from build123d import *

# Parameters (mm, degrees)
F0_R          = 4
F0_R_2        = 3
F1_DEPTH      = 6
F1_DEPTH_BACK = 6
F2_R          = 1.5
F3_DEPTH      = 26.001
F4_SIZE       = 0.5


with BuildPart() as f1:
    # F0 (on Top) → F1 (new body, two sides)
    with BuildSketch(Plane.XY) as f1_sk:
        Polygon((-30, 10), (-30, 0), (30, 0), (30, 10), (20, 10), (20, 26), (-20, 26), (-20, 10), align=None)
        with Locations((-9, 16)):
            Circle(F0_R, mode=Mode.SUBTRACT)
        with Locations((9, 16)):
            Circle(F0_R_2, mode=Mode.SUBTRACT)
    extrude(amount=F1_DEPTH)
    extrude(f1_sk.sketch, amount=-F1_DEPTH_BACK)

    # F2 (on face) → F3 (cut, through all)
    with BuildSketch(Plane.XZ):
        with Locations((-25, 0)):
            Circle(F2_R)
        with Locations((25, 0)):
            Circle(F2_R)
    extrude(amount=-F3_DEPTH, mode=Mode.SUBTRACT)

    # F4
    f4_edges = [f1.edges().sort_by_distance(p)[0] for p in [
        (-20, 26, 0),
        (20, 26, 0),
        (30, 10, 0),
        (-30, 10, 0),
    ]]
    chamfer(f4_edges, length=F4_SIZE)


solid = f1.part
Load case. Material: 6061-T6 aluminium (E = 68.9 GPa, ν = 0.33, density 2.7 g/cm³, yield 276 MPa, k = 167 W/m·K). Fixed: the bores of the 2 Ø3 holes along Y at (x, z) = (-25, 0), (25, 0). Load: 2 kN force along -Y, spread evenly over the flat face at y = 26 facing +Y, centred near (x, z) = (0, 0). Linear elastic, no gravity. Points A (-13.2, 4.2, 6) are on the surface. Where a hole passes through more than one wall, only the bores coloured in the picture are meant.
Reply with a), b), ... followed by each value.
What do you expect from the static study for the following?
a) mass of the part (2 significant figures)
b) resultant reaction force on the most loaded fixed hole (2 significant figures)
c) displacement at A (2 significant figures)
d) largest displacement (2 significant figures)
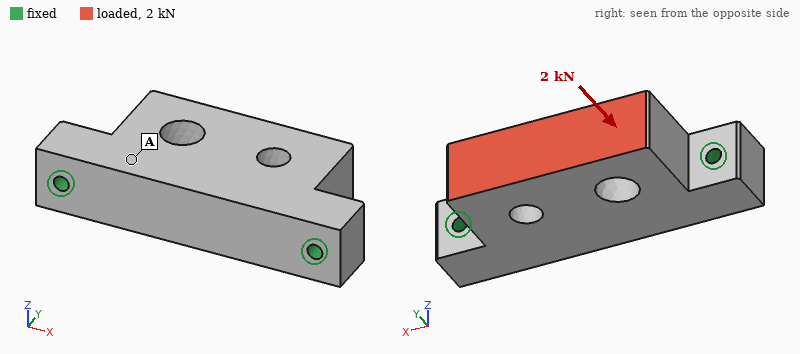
a) 37 g
b) 1.1 kN
c) 5.2 µm
d) 7.7 µm
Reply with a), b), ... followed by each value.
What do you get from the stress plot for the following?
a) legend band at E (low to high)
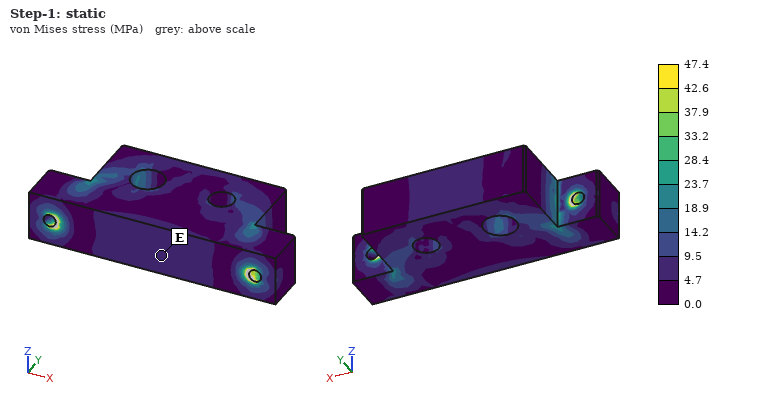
a) 4.7 to 9.5 MPa
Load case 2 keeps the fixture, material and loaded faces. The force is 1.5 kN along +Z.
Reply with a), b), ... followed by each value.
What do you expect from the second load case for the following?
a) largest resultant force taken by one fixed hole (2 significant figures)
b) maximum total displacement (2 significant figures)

a) 750 N
b) 84 µm
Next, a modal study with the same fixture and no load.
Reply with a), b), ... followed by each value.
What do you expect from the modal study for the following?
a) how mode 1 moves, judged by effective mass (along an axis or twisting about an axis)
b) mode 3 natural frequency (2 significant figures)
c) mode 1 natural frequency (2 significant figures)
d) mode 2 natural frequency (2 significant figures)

a) along Z
b) 16 kHz
c) 7200 Hz
d) 16 kHz
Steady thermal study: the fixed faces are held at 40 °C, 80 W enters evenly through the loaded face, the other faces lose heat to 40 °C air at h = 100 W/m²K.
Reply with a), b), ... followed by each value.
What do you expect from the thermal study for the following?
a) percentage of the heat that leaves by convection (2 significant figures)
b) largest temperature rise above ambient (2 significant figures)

a) 11 %
b) 41 K
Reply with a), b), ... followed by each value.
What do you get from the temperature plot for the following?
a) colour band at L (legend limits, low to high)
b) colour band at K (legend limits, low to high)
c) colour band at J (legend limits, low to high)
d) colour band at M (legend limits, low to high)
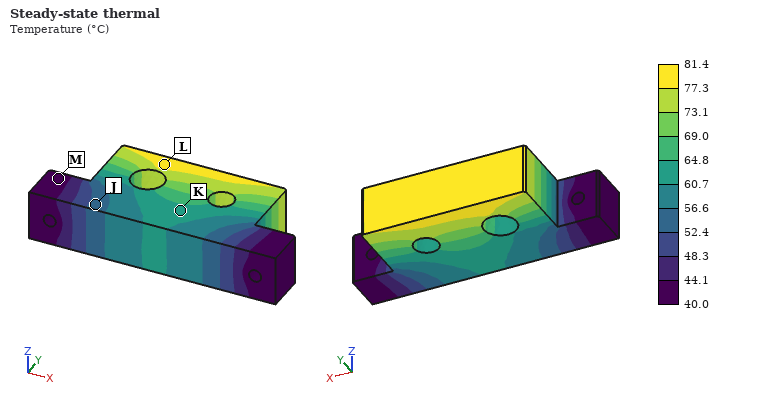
a) 77.3 to 81.4 °C
b) 60.7 to 64.8 °C
c) 52.4 to 56.6 °C
d) 40.0 to 44.1 °C
